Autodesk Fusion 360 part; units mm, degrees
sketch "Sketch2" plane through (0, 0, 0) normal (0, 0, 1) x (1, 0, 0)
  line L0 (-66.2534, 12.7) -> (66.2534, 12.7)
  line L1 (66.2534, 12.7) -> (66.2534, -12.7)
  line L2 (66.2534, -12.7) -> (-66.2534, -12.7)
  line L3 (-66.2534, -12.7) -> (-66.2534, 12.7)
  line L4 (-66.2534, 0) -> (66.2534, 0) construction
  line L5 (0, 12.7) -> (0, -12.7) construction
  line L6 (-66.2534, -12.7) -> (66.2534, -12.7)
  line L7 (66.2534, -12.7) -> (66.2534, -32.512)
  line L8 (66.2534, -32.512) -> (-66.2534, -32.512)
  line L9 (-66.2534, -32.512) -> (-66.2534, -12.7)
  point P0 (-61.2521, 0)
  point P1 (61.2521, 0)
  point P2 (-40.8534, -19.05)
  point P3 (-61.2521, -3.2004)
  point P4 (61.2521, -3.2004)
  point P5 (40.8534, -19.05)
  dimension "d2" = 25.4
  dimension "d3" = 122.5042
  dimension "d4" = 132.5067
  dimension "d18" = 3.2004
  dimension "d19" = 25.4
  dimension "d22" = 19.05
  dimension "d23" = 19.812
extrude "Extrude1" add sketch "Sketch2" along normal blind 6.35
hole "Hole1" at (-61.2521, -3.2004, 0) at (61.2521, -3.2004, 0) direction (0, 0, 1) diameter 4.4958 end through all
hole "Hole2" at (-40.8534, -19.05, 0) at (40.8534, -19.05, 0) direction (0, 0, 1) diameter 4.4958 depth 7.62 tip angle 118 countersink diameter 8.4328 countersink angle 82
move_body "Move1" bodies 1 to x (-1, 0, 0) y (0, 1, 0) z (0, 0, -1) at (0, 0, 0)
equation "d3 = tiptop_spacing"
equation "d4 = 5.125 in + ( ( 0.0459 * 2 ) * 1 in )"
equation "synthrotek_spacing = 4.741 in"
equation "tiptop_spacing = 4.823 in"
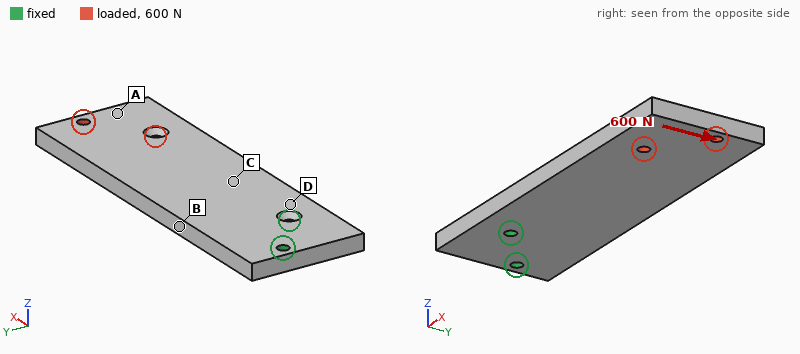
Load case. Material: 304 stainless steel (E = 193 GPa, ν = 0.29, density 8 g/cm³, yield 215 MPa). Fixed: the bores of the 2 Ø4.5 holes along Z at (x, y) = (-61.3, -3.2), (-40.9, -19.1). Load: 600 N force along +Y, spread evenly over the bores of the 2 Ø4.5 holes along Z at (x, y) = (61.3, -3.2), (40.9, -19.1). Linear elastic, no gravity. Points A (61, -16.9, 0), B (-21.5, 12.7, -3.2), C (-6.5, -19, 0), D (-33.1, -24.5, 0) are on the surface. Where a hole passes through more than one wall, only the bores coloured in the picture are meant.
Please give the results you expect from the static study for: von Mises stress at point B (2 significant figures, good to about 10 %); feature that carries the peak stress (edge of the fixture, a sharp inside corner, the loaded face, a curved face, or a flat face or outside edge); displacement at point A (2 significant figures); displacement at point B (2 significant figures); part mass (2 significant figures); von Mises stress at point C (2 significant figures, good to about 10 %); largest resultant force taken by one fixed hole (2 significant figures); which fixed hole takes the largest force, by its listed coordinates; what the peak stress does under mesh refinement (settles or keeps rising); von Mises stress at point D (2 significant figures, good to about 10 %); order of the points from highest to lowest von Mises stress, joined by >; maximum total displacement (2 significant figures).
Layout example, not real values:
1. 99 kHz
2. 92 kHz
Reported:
1. 22 MPa
2. edge of the fixture
3. 39 µm
4. 8.7 µm
5. 300 g
6. 7.7 MPa
7. 2.4 kN
8. (-40.9, -19.1)
9. keeps rising
10. 16 MPa
11. B > D > C > A
12. 43 µm
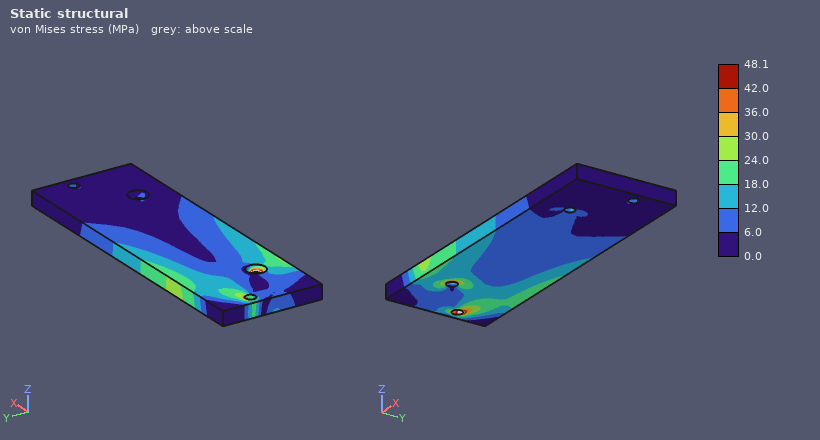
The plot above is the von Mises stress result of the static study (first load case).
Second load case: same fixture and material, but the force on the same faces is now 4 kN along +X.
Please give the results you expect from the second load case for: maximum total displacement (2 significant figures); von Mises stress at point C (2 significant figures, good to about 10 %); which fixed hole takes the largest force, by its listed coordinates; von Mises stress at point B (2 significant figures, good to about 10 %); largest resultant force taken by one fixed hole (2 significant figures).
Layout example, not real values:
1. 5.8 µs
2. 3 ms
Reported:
1. 51 µm
2. 8.0 MPa
3. (-40.9, -19.1)
4. 15 MPa
5. 2.3 kN
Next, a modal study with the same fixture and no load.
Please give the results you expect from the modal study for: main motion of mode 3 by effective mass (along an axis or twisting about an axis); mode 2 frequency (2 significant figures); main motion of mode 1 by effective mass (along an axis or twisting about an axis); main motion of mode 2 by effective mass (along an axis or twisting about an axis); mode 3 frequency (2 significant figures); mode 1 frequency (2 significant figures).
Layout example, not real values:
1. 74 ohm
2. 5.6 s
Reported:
1. along Y
2. 1800 Hz
3. along Z
4. twisting about X
5. 2100 Hz
6. 400 Hz
